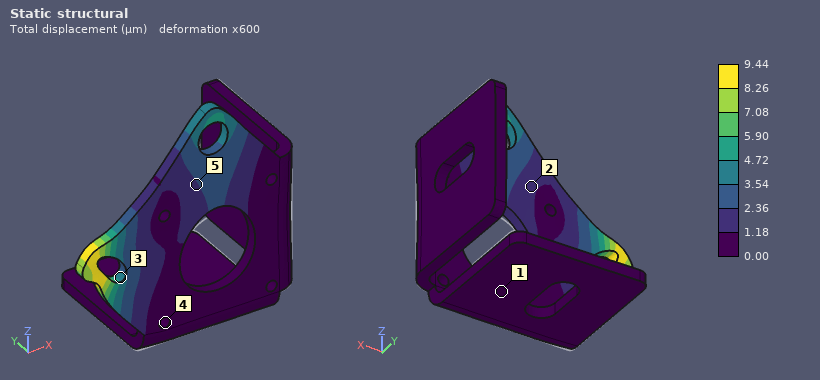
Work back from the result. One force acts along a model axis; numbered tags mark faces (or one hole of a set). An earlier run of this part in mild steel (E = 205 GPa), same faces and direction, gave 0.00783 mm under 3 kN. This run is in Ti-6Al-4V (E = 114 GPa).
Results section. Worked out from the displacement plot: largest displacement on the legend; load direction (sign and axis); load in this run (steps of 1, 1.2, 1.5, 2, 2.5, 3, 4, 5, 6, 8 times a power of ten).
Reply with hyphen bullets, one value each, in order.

- 9.44 µm
- +Z
- 2 kN
